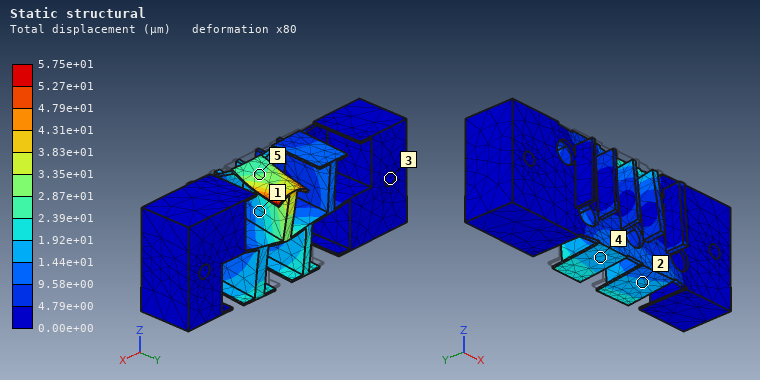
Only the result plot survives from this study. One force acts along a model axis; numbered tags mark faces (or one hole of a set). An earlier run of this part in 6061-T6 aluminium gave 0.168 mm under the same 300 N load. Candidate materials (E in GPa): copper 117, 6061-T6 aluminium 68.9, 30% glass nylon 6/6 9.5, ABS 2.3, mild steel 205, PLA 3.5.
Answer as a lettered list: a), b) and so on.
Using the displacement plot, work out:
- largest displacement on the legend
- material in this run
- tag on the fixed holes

a) 5.75e+01 µm
b) mild steel
c) 3
